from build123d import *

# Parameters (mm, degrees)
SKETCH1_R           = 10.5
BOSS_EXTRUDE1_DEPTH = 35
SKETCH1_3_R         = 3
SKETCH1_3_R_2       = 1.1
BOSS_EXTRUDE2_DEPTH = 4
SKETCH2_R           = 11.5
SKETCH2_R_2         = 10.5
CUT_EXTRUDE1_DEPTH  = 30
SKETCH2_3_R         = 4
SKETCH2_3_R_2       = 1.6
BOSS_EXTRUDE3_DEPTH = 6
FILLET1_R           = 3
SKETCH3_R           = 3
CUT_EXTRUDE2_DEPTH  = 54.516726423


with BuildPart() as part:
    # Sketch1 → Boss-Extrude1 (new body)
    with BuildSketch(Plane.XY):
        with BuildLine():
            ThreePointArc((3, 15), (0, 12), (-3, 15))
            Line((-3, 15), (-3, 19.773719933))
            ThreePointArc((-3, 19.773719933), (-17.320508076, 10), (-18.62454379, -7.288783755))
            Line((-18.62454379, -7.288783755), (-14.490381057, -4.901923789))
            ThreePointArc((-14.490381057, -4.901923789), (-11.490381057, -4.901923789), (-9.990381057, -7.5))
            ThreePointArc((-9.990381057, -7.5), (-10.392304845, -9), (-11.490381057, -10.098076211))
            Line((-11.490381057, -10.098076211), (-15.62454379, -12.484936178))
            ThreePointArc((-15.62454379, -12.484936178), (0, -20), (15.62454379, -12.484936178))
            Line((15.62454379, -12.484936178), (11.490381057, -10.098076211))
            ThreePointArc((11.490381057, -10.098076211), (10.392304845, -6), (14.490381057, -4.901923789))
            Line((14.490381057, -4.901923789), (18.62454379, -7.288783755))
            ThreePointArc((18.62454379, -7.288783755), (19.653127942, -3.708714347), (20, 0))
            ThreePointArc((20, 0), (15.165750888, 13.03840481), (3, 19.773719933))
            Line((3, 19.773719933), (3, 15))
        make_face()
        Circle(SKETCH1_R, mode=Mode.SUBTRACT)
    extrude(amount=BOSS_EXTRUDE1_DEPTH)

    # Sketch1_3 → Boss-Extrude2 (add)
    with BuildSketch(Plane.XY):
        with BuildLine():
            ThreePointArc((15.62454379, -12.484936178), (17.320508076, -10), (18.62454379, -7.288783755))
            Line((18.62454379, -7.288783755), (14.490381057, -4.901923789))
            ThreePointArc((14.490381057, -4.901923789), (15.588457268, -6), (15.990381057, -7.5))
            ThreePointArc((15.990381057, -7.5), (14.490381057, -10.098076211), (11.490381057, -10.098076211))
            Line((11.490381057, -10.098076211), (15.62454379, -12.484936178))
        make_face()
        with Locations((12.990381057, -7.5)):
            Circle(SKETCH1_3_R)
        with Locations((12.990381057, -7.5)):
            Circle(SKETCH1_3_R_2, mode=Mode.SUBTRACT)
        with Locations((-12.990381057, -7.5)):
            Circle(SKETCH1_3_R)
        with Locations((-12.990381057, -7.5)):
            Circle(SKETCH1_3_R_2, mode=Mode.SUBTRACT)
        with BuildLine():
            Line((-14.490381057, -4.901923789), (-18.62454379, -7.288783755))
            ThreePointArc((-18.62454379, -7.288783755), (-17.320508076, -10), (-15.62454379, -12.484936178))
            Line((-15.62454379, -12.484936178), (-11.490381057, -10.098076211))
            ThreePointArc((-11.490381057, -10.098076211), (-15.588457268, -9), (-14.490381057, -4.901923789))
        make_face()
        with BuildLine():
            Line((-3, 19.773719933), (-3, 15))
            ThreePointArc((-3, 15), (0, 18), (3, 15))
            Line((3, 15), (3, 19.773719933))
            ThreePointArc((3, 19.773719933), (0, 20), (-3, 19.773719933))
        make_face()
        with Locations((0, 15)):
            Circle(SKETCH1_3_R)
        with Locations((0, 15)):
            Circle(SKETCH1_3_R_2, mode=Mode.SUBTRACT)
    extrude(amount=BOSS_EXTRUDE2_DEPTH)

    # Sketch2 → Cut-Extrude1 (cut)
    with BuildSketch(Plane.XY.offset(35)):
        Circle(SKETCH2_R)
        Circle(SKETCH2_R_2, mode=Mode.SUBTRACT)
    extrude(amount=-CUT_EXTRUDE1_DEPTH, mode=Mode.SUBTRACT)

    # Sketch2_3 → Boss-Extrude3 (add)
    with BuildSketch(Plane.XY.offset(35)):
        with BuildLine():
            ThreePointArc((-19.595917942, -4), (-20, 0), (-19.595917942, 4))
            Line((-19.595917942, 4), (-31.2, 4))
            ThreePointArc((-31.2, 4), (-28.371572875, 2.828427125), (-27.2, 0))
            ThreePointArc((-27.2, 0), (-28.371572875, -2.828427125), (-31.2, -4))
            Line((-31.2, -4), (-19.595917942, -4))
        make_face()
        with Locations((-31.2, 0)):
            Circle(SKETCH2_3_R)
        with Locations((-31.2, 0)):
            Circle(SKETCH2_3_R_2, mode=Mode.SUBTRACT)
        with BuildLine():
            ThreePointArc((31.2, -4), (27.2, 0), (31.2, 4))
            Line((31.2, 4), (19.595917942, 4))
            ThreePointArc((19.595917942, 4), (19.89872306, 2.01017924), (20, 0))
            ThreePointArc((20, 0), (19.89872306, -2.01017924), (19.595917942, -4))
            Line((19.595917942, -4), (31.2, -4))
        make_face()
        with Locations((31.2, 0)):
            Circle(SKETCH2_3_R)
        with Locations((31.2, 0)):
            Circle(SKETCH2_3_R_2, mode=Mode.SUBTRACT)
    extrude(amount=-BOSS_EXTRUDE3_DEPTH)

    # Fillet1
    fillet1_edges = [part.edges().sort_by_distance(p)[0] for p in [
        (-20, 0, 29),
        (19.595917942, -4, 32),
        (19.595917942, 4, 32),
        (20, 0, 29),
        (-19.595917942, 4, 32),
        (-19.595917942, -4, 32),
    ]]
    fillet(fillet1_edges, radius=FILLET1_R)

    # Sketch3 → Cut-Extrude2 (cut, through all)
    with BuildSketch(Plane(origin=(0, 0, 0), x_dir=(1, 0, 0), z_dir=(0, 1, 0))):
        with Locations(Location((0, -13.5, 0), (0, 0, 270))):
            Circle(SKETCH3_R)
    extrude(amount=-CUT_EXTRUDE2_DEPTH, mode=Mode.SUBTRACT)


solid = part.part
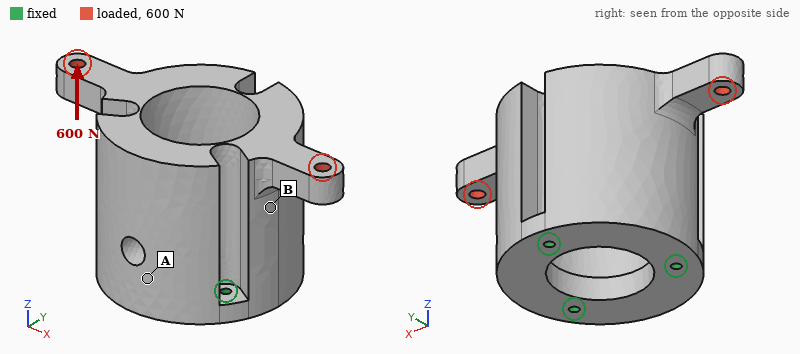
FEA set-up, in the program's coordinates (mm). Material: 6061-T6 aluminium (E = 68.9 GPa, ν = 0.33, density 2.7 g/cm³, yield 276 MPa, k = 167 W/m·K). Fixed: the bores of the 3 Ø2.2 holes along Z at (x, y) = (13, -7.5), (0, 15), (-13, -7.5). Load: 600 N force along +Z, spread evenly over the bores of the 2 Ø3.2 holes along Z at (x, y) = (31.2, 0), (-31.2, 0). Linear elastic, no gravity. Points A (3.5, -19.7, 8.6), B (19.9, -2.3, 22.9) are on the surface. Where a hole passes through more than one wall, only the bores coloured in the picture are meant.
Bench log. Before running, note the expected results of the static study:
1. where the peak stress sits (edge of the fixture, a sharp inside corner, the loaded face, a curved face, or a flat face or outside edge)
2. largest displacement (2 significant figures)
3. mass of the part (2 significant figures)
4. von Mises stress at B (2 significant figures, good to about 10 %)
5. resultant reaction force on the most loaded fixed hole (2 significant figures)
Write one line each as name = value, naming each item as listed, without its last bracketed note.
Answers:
where the peak stress sits = a curved face
largest displacement = 49 µm
mass of the part = 72 g
von Mises stress at B = 15 MPa
resultant reaction force on the most loaded fixed hole = 220 N
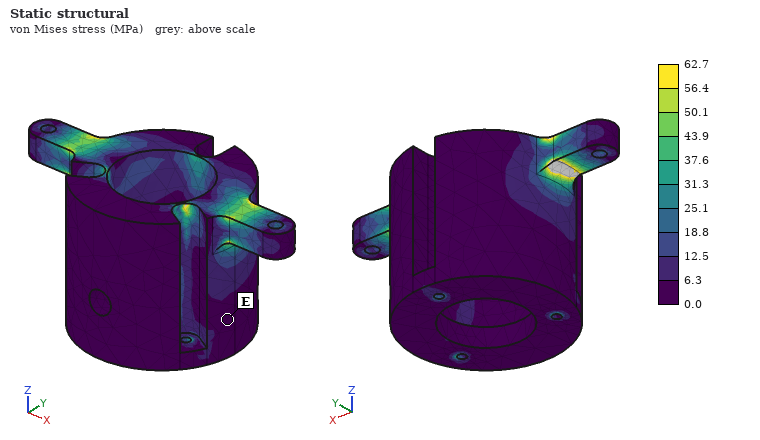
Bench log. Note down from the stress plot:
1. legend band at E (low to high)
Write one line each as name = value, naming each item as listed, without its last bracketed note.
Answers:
legend band at E = 0.0 to 6.3 MPa
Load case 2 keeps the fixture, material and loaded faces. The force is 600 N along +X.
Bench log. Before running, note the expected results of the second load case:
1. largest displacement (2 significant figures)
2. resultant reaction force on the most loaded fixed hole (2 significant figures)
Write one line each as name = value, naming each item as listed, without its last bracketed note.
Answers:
largest displacement = 26 µm
resultant reaction force on the most loaded fixed hole = 670 N
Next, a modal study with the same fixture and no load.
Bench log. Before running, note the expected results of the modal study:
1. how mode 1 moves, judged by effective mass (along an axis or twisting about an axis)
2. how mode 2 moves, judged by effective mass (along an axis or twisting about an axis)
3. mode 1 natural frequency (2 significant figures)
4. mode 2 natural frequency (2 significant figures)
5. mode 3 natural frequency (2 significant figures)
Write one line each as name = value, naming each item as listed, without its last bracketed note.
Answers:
how mode 1 moves, judged by effective mass = along X
how mode 2 moves, judged by effective mass = along Y
mode 1 natural frequency = 5900 Hz
mode 2 natural frequency = 6200 Hz
mode 3 natural frequency = 10 kHz
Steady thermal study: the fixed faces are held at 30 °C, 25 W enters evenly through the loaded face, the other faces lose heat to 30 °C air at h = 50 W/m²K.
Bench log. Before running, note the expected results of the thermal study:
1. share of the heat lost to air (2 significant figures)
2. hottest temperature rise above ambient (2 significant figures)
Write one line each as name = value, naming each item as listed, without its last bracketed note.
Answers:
share of the heat lost to air = 16 %
hottest temperature rise above ambient = 35 K
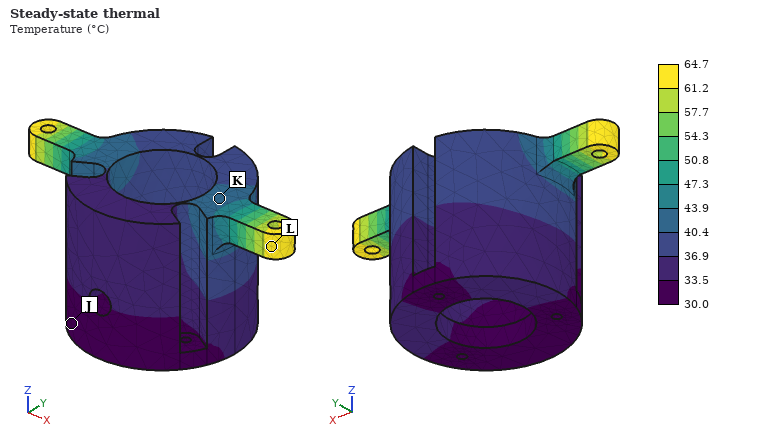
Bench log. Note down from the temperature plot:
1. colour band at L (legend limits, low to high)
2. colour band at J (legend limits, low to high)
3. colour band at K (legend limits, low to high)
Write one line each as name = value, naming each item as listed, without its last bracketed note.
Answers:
colour band at L = 61.2 to 64.7 °C
colour band at J = 30.0 to 33.5 °C
colour band at K = 40.4 to 43.9 °C
